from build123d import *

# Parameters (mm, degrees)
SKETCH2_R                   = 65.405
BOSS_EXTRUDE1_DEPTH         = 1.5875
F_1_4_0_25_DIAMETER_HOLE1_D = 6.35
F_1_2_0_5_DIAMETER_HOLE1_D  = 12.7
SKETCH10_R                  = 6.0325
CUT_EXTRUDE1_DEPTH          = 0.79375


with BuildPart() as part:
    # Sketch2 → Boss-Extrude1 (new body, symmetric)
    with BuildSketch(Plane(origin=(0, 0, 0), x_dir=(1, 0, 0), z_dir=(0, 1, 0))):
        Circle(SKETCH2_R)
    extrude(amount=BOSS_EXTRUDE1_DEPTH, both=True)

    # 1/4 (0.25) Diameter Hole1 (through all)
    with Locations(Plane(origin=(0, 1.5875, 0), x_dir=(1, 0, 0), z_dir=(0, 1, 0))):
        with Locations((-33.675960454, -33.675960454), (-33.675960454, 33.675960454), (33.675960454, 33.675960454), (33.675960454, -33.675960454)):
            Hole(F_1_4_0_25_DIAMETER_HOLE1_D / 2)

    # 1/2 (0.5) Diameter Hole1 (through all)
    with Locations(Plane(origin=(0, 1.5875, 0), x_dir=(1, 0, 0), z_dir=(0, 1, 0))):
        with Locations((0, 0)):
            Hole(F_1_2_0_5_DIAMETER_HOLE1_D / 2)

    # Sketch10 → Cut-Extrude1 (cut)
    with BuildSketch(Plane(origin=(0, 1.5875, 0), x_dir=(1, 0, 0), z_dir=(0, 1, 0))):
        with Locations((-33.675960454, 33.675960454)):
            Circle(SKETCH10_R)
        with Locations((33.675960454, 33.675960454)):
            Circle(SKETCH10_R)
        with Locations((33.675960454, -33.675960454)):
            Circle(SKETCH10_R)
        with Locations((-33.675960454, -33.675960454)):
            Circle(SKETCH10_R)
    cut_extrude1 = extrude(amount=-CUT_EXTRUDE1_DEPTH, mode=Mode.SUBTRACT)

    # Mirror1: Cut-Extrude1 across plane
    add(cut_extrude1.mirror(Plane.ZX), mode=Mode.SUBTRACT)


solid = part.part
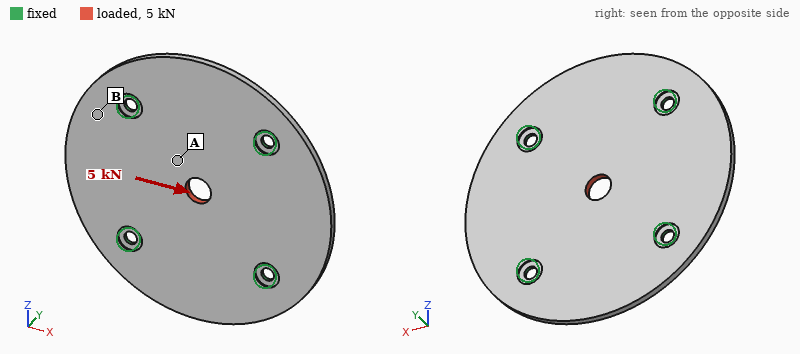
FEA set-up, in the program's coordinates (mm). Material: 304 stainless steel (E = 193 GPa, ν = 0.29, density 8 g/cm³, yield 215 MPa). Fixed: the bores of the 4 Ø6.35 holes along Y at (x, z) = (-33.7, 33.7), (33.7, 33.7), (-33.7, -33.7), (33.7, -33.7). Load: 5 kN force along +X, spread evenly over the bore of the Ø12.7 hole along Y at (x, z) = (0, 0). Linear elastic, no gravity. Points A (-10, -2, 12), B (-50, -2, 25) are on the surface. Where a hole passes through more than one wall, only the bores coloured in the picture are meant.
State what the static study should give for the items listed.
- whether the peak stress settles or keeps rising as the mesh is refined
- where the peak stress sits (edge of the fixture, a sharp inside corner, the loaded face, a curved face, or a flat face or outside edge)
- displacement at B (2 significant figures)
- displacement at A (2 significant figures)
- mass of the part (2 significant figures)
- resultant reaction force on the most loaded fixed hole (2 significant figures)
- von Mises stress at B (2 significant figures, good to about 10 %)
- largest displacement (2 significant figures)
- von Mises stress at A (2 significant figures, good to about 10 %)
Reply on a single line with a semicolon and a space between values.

keeps rising; edge of the fixture; 1.6 µm; 3.7 µm; 330 g; 1.3 kN; 7.7 MPa; 6.0 µm; 21 MPa
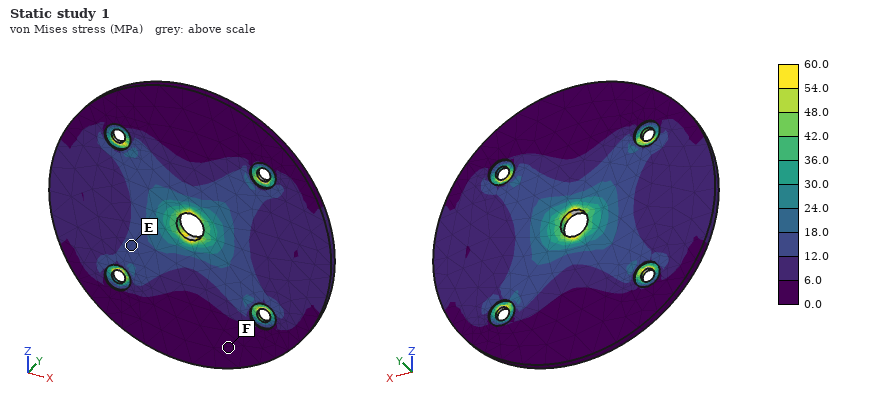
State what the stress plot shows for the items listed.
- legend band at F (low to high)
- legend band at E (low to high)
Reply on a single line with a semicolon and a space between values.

0.0 to 6.0 MPa; 12.0 to 18.0 MPa
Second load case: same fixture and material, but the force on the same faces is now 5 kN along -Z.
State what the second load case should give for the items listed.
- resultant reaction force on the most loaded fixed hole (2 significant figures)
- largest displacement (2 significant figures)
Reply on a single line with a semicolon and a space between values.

1.3 kN; 6.0 µm
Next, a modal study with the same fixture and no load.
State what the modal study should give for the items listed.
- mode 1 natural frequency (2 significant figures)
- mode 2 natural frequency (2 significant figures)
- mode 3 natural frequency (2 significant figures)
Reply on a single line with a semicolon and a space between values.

1600 Hz; 1800 Hz; 1800 Hz
